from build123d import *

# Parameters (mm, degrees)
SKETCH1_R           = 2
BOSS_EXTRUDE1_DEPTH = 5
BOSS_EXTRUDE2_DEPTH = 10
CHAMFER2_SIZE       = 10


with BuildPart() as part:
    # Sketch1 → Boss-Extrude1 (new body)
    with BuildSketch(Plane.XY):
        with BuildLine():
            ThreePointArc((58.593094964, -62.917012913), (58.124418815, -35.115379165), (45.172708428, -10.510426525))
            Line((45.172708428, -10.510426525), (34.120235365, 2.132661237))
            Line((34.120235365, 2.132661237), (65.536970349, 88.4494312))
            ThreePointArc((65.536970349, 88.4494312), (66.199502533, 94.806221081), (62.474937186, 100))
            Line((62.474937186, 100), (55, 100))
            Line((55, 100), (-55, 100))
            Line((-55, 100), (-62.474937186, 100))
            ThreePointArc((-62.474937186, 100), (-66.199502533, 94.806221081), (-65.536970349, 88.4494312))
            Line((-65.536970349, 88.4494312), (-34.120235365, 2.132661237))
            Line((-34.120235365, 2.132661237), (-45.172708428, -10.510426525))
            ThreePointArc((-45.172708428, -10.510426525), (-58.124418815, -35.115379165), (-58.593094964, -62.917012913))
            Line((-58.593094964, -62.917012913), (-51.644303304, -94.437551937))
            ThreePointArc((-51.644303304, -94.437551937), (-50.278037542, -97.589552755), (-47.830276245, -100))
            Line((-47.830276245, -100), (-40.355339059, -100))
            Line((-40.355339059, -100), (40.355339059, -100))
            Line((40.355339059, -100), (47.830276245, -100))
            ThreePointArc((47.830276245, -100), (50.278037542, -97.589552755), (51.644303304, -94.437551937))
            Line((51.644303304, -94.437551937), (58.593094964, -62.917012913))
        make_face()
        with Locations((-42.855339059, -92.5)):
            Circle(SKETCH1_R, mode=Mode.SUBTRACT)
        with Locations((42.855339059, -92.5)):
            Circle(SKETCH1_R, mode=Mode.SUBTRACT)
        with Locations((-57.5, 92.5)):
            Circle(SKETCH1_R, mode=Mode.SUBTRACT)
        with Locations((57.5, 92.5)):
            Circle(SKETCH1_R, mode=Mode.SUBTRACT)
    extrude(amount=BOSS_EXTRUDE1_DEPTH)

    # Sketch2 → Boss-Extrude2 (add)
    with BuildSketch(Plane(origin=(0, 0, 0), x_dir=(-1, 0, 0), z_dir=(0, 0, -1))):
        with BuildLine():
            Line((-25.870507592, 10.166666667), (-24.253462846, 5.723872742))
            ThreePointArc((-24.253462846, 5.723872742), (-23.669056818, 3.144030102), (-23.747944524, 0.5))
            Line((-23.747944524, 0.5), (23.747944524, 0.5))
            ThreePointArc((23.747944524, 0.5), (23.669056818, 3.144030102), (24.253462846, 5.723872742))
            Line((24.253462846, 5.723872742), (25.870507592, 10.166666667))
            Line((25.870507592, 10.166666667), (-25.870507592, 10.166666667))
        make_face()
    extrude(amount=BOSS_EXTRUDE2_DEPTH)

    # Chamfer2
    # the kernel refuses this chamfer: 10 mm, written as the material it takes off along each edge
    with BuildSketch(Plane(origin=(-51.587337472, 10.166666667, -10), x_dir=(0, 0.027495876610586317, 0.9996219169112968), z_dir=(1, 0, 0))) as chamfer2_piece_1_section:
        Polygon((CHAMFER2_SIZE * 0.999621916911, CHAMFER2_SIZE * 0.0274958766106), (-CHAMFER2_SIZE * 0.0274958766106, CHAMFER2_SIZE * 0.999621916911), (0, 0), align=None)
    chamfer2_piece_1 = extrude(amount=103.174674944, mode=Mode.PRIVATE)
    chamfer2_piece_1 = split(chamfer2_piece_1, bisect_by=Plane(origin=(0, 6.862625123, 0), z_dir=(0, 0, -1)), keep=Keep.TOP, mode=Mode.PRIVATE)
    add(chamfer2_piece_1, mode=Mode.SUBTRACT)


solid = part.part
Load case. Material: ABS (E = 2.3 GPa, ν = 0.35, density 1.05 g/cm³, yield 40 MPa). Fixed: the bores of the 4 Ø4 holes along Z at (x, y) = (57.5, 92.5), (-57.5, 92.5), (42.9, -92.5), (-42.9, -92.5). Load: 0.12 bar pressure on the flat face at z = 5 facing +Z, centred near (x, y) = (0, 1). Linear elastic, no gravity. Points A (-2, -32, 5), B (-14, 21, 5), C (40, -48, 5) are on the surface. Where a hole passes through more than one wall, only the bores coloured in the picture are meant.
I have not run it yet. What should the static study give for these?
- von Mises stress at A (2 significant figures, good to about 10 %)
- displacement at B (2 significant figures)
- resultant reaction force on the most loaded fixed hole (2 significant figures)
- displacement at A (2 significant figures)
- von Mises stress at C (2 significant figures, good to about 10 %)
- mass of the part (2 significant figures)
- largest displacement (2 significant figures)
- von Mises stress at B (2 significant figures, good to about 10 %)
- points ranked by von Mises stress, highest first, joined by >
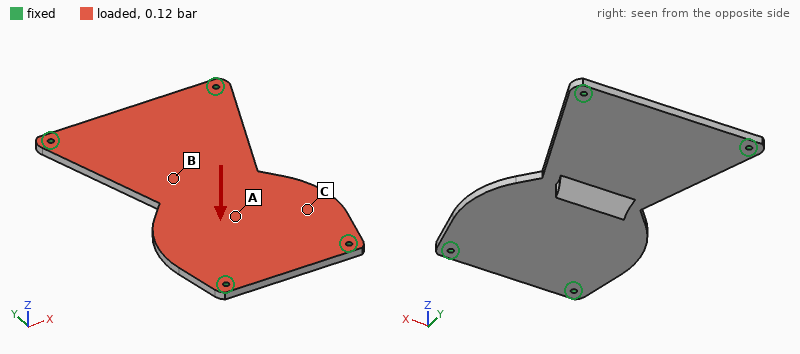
3.0 MPa
2.3 mm
64 N
1.9 mm
1.4 MPa
110 g
2.4 mm
4.7 MPa
B > A > C
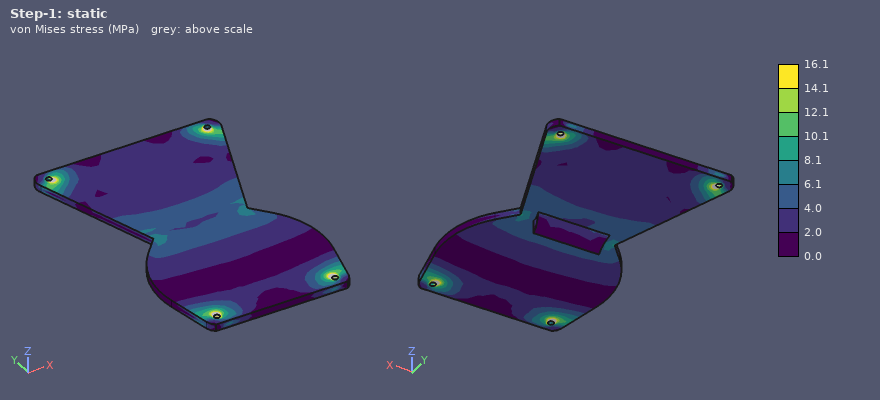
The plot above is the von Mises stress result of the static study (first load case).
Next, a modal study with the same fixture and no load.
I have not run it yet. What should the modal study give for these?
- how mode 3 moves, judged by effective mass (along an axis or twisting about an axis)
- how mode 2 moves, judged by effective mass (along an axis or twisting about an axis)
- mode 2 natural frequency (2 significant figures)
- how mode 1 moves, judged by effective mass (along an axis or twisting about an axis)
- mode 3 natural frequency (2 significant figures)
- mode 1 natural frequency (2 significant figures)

twisting about X
twisting about Y
370 Hz
along Z
450 Hz
180 Hz
